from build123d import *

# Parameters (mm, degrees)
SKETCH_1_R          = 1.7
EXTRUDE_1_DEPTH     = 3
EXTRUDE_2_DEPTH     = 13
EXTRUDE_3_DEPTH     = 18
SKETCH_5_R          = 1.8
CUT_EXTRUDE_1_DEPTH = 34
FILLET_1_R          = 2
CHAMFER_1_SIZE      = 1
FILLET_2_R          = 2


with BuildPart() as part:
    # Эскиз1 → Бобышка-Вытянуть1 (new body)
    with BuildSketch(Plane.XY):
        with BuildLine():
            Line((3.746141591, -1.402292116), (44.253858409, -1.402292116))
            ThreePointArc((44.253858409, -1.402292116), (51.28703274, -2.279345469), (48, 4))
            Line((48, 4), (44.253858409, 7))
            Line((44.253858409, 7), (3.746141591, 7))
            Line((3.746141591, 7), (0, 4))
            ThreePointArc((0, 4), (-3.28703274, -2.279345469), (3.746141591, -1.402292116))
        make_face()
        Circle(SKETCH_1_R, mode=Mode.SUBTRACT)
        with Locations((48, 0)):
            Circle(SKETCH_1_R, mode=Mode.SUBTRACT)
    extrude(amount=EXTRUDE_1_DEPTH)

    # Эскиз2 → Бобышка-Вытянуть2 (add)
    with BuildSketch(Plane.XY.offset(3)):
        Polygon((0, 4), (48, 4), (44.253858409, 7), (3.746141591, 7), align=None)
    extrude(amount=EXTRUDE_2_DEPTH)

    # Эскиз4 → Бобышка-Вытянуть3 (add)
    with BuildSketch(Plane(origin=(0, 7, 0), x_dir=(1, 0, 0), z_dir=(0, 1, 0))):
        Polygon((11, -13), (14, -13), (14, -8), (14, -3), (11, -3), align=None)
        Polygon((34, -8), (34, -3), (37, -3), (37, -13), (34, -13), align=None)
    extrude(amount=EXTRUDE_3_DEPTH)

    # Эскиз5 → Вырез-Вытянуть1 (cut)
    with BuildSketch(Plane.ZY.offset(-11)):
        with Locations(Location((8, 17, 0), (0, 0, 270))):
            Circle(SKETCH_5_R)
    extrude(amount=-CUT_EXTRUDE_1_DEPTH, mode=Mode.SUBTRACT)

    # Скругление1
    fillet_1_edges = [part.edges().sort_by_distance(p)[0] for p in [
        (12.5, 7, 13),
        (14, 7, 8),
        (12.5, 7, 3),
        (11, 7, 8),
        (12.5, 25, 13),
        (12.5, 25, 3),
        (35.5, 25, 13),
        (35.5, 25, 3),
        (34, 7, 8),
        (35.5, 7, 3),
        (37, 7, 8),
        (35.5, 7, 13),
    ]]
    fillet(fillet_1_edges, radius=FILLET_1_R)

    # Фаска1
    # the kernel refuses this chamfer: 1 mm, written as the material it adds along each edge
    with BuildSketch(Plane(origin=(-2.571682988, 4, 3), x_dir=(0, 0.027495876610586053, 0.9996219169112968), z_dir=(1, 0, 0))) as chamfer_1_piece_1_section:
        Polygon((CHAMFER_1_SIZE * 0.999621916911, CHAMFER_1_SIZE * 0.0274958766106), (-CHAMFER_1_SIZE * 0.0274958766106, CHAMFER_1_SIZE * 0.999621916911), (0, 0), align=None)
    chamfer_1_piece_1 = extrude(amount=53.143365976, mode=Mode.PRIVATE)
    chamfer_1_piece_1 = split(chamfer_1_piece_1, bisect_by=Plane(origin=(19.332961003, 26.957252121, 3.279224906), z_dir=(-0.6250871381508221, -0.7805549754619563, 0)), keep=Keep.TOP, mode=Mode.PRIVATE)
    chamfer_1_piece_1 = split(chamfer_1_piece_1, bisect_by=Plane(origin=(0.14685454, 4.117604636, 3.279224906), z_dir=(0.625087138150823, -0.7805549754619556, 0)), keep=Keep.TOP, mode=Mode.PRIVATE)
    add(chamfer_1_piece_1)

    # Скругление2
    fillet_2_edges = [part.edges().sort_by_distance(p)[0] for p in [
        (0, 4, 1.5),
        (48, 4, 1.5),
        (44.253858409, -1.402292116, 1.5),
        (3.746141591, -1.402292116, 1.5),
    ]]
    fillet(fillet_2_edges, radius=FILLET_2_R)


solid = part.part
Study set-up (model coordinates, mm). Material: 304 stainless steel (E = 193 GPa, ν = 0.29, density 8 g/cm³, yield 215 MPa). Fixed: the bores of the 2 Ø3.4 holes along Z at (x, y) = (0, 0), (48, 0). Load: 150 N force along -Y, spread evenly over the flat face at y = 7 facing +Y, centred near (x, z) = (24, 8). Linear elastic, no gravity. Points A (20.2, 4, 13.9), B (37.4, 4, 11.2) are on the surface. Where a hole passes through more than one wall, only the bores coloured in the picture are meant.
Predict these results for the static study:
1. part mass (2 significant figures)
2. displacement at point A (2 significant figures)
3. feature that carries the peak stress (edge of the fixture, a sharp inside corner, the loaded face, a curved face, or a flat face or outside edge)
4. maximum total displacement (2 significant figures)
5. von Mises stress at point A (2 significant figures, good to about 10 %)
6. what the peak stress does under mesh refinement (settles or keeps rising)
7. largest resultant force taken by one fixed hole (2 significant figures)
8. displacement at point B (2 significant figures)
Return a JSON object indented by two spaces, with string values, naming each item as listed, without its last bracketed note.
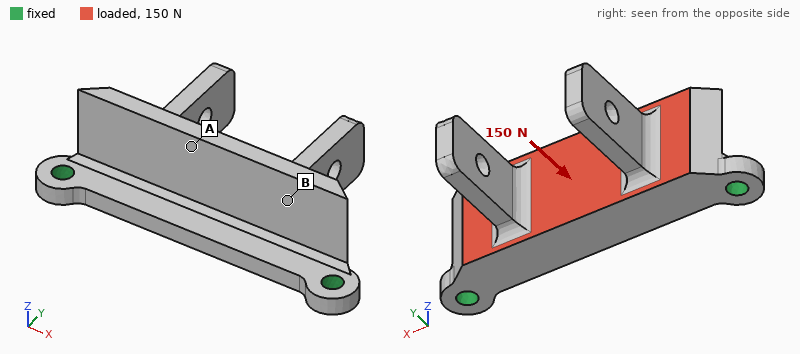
{
  "part mass": "33 g",
  "displacement at point A": "14 µm",
  "feature that carries the peak stress": "edge of the fixture",
  "maximum total displacement": "23 µm",
  "von Mises stress at point A": "8.7 MPa",
  "what the peak stress does under mesh refinement": "keeps rising",
  "largest resultant force taken by one fixed hole": "99 N",
  "displacement at point B": "9.6 µm"
}
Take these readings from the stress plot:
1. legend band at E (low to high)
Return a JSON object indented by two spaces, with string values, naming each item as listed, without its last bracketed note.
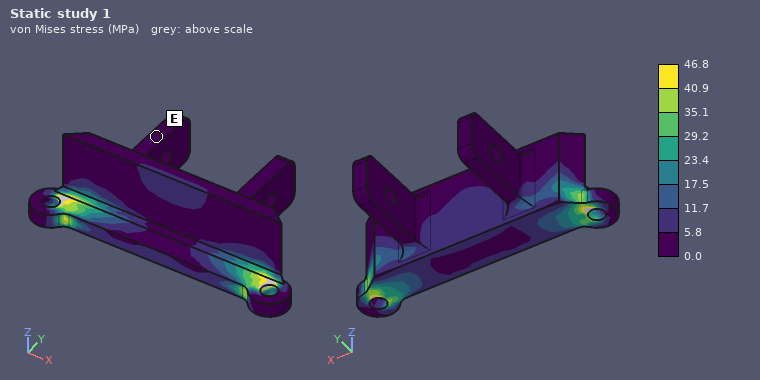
{
  "legend band at E": "0.0 to 5.8 MPa"
}
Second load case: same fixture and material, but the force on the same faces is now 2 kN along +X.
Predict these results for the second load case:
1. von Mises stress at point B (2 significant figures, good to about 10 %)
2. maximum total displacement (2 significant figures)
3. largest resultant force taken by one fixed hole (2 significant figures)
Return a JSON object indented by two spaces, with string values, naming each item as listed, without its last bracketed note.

{
  "von Mises stress at point B": "11 MPa",
  "maximum total displacement": "6.0 µm",
  "largest resultant force taken by one fixed hole": "1.1 kN"
}
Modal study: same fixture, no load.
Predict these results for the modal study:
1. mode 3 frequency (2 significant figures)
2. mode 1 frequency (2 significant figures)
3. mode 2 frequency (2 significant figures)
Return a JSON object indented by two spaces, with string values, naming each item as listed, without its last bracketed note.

{
  "mode 3 frequency": "6300 Hz",
  "mode 1 frequency": "2800 Hz",
  "mode 2 frequency": "6200 Hz"
}
